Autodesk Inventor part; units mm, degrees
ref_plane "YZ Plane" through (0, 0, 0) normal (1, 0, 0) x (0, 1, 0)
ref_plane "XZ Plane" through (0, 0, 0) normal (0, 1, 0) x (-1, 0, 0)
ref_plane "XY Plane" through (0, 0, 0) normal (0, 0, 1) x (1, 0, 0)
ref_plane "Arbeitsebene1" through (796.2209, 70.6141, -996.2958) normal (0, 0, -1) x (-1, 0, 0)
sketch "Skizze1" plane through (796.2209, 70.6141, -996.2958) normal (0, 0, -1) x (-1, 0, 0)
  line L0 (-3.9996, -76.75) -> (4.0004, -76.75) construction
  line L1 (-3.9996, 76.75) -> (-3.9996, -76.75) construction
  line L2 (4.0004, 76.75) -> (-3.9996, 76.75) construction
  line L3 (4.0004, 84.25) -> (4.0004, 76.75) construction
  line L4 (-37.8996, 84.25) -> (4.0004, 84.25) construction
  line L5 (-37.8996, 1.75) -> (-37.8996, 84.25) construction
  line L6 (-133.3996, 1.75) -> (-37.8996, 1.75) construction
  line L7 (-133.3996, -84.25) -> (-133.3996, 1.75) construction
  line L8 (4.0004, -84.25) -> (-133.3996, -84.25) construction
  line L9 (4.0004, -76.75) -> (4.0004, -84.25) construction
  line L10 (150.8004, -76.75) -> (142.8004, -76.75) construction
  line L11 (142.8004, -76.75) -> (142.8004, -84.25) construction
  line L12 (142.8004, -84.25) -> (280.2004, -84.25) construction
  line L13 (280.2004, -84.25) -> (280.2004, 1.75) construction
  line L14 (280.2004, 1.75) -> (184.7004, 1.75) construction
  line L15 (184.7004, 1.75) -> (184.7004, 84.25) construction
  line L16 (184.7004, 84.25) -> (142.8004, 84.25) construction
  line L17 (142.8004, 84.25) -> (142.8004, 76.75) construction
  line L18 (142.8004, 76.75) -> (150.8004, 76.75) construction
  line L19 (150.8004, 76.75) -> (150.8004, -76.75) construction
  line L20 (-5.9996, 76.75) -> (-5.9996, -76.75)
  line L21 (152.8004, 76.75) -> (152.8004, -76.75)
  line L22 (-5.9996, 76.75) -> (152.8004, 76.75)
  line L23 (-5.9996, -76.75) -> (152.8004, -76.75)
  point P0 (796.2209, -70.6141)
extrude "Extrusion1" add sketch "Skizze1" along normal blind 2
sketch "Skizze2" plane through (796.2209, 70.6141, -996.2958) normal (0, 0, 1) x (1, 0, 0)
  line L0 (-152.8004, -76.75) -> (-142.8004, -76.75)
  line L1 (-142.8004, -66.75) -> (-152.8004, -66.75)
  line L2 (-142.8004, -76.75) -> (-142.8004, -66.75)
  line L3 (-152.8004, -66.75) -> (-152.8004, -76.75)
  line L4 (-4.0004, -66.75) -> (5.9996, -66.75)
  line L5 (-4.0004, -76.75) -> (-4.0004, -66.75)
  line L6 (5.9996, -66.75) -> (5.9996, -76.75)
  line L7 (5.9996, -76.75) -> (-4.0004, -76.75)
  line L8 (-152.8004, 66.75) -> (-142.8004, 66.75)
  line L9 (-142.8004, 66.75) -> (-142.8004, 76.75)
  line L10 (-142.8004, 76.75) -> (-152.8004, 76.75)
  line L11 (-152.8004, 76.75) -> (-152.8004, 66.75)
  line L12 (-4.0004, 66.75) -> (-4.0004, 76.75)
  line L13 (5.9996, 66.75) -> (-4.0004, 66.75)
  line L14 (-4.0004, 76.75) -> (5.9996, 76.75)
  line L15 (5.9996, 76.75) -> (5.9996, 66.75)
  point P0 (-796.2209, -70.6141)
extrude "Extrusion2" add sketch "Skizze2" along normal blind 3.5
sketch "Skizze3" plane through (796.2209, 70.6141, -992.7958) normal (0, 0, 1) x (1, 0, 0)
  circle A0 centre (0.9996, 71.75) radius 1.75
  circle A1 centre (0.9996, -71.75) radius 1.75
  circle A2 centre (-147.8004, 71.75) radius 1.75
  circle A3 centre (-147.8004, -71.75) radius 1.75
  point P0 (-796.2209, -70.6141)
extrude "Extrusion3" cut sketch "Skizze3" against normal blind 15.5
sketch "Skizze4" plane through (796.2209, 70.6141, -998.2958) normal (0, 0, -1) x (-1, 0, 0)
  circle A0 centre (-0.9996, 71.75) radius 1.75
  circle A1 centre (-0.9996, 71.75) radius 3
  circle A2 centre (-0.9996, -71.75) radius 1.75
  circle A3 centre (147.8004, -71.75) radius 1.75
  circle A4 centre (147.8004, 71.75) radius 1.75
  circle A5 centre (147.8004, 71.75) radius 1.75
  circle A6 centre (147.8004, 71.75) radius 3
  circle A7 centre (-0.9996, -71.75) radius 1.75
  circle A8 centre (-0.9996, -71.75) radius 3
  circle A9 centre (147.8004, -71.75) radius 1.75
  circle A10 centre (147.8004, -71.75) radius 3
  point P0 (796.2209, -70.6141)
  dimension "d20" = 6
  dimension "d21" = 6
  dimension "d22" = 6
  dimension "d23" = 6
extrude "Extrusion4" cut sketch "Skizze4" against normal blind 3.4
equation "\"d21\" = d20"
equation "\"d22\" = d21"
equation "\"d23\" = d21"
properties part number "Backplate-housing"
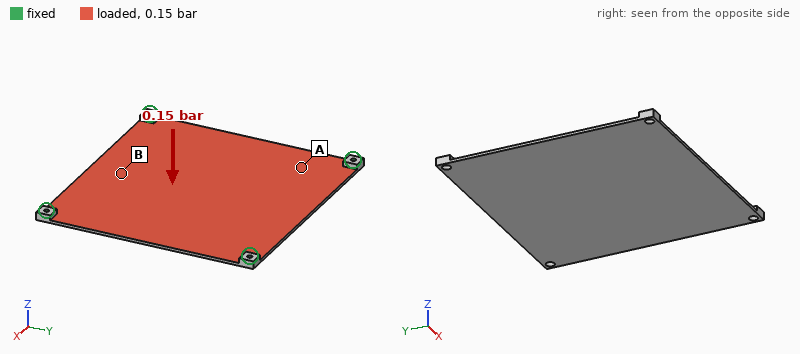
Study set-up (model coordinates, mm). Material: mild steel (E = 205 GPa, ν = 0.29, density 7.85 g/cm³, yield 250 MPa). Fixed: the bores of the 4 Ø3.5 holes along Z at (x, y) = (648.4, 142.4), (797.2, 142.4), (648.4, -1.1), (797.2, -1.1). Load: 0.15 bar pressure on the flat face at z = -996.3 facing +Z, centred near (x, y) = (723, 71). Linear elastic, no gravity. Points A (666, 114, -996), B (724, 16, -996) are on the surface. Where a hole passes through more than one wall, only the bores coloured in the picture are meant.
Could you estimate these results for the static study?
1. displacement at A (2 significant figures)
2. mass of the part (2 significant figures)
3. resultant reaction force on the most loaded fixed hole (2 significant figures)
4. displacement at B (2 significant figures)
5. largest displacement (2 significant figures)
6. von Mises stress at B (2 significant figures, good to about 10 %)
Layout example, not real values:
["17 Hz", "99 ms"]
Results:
["0.13 mm", "390 g", "330 N", "0.26 mm", "0.36 mm", "26 MPa"]
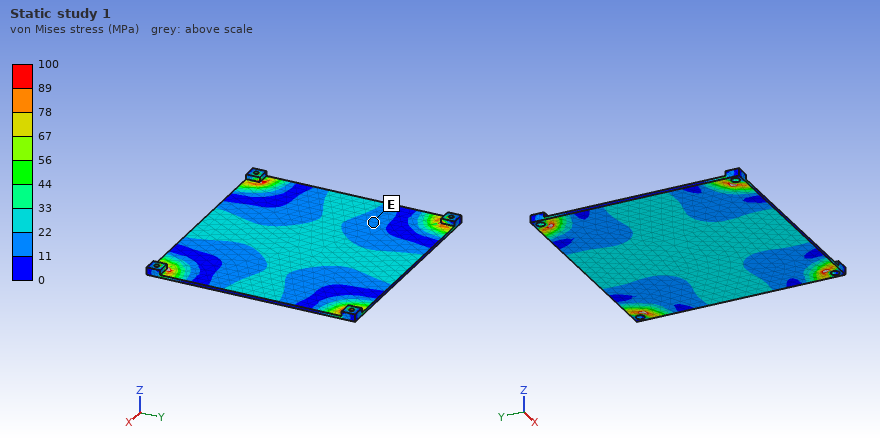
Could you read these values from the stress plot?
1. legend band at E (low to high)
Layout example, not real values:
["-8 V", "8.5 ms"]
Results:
["11 to 22 MPa"]
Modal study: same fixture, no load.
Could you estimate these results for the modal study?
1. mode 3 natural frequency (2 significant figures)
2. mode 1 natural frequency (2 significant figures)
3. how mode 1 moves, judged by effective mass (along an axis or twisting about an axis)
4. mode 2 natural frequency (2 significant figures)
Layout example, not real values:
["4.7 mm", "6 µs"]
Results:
["570 Hz", "310 Hz", "along Z", "550 Hz"]
